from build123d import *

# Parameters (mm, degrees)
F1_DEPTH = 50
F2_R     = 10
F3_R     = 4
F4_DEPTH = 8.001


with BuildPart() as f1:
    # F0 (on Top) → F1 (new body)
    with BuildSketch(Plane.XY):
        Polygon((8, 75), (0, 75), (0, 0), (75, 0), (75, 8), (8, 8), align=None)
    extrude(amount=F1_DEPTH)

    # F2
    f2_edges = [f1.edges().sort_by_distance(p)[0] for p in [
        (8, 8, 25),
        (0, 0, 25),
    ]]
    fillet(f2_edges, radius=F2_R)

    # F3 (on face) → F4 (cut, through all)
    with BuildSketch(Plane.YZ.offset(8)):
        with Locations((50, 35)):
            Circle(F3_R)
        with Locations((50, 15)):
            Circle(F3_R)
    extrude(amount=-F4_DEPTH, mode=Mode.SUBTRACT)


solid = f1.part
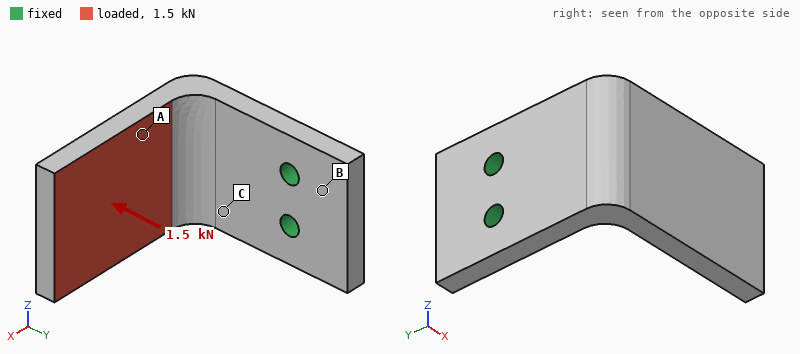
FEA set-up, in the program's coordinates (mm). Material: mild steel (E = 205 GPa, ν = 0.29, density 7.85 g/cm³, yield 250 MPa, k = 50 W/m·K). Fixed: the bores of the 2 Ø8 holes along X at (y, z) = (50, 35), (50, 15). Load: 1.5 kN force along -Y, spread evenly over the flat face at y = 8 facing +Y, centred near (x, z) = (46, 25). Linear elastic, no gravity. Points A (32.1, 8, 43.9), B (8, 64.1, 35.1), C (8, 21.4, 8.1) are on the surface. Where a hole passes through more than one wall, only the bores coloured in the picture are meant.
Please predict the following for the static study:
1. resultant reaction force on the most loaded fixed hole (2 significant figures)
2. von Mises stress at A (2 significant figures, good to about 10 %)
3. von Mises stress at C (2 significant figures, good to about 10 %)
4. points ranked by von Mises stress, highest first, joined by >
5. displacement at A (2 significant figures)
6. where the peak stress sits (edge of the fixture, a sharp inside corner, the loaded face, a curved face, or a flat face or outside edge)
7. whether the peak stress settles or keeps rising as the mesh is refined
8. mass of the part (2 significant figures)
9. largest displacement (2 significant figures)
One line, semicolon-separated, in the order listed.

770 N; 45 MPa; 120 MPa; C > A > B; 0.20 mm; edge of the fixture; keeps rising; 440 g; 0.54 mm
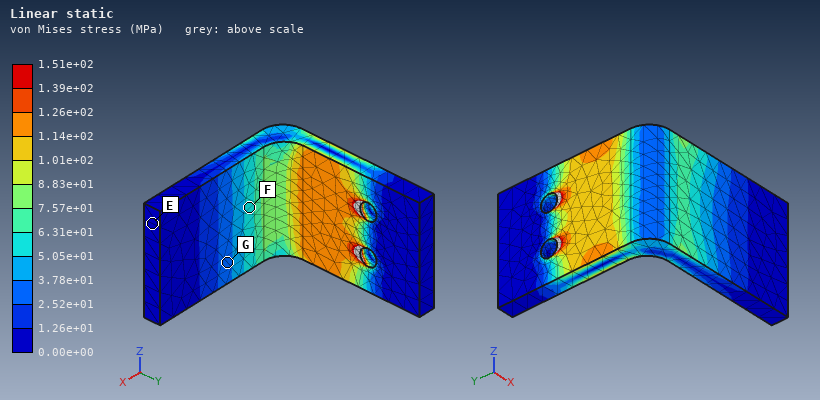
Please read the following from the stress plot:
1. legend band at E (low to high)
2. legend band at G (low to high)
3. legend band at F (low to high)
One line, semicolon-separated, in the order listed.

0.00e+00 to 1.26e+01 MPa; 2.52e+01 to 3.78e+01 MPa; 5.05e+01 to 6.31e+01 MPa
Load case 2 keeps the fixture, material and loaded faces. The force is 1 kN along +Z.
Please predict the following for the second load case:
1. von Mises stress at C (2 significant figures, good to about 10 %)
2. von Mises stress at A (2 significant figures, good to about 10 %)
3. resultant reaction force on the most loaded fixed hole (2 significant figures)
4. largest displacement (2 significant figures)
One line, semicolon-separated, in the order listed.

55 MPa; 14 MPa; 2.1 kN; 0.14 mm
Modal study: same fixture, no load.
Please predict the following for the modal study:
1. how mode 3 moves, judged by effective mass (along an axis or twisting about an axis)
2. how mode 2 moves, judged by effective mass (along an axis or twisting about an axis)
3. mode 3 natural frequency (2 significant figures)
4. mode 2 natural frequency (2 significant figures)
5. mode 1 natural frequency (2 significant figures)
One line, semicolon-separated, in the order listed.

along X; along Z; 2200 Hz; 1200 Hz; 690 Hz
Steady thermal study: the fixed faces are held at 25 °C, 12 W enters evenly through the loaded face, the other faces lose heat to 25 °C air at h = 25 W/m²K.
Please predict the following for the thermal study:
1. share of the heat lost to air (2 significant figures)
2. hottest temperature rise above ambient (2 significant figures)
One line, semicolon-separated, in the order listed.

39 %; 32 K
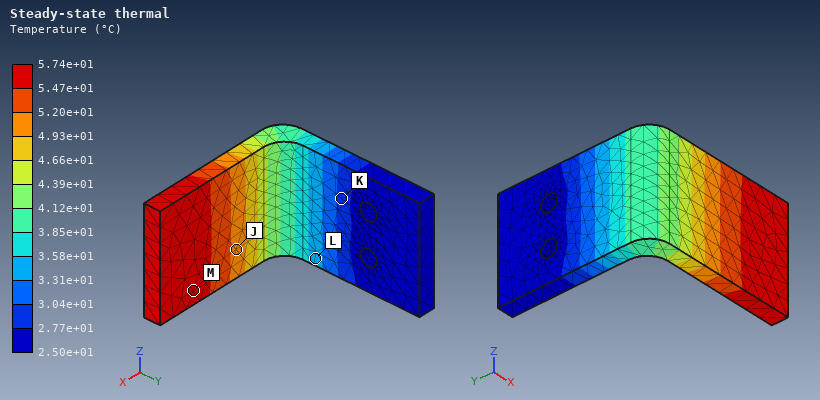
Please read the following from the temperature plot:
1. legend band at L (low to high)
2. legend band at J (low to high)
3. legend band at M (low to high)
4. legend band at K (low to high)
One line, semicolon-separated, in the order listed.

3.31e+01 to 3.58e+01 °C; 4.93e+01 to 5.20e+01 °C; 5.47e+01 to 5.74e+01 °C; 2.77e+01 to 3.04e+01 °C
